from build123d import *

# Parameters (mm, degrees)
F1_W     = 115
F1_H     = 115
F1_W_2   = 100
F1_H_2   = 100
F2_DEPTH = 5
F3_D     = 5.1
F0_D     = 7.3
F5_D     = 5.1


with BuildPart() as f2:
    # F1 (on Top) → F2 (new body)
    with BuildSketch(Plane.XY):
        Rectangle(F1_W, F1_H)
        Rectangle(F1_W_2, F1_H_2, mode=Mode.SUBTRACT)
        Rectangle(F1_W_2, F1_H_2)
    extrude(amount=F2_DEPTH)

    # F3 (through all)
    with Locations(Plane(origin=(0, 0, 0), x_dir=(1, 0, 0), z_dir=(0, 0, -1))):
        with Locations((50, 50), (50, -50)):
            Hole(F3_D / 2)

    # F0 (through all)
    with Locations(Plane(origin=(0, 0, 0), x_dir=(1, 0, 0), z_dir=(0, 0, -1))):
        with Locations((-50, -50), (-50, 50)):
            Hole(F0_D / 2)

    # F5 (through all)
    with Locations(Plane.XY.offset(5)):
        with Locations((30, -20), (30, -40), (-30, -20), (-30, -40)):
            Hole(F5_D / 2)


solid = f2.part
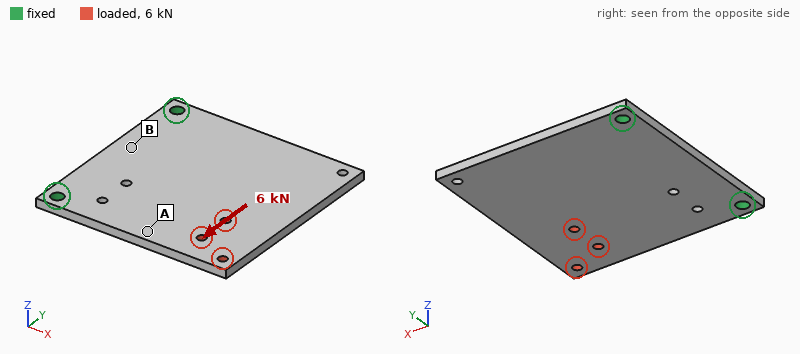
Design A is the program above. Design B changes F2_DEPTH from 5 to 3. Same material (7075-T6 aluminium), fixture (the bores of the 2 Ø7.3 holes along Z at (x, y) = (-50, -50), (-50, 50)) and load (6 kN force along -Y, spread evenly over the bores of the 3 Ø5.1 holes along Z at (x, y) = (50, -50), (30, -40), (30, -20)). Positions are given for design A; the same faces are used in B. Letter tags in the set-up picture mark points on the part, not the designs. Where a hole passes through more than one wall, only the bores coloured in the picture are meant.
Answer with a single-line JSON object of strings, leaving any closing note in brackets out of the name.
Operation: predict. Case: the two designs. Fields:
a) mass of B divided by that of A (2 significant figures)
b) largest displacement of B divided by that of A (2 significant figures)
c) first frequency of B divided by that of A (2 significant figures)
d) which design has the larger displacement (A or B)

{"mass of B divided by that of A": "0.60", "largest displacement of B divided by that of A": "1.7", "first frequency of B divided by that of A": "0.61", "which design has the larger displacement": "B"}
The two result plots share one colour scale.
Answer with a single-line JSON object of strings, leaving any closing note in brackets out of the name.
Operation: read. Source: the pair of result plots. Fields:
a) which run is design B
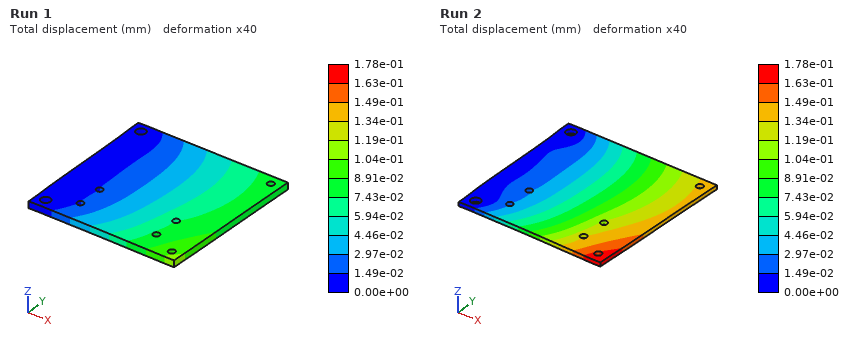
{"which run is design B": "Run 2"}
